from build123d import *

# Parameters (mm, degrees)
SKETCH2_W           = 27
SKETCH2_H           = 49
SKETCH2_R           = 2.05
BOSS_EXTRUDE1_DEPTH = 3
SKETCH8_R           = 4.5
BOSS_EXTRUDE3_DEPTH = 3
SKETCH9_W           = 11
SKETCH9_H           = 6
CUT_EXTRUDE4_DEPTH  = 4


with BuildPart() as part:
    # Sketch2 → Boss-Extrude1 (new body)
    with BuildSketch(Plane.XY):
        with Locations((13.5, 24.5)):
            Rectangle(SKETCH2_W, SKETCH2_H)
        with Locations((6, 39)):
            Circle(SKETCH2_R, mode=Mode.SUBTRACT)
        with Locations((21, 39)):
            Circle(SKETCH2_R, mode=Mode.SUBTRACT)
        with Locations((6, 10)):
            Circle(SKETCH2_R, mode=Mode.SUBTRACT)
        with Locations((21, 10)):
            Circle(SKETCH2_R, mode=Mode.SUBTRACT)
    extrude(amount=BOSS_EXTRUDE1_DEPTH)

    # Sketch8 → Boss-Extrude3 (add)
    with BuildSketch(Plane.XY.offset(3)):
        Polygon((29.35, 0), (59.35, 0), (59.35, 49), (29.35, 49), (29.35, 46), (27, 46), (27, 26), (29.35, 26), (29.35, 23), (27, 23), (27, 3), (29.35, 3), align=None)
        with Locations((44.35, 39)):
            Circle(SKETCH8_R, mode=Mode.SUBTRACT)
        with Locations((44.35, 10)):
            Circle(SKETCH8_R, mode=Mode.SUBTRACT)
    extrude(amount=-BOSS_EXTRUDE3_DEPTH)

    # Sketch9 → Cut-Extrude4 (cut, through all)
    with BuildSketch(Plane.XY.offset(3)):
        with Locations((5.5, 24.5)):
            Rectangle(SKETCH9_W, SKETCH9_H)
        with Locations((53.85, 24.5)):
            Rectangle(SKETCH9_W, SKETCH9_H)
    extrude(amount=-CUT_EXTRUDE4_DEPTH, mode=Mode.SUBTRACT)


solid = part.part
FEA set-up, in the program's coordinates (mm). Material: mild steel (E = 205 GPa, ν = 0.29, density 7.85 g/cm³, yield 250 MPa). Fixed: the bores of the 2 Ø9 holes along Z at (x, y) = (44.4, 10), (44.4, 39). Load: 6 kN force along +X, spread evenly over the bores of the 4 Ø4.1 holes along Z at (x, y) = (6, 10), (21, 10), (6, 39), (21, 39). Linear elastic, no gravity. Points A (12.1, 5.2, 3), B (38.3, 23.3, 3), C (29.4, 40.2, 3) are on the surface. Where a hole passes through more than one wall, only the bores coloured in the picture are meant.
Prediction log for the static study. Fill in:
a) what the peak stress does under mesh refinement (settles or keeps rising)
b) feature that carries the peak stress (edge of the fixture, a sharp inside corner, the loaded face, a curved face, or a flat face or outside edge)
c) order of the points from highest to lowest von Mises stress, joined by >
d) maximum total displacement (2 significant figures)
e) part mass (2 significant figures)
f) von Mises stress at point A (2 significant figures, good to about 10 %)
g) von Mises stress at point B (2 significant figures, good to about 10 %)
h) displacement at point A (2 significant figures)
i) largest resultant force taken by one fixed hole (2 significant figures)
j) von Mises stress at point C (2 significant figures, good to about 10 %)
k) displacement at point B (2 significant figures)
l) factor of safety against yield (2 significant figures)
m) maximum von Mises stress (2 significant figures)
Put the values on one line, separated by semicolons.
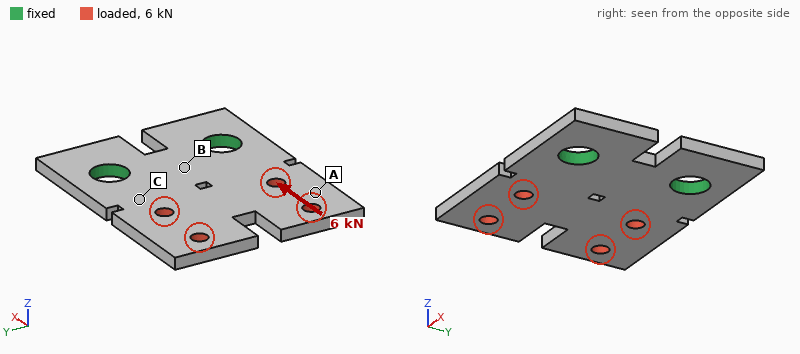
settles; the loaded face; C > A > B; 9.5 µm; 61 g; 33 MPa; 16 MPa; 7.6 µm; 3.0 kN; 52 MPa; 1.9 µm; 1.7; 150 MPa
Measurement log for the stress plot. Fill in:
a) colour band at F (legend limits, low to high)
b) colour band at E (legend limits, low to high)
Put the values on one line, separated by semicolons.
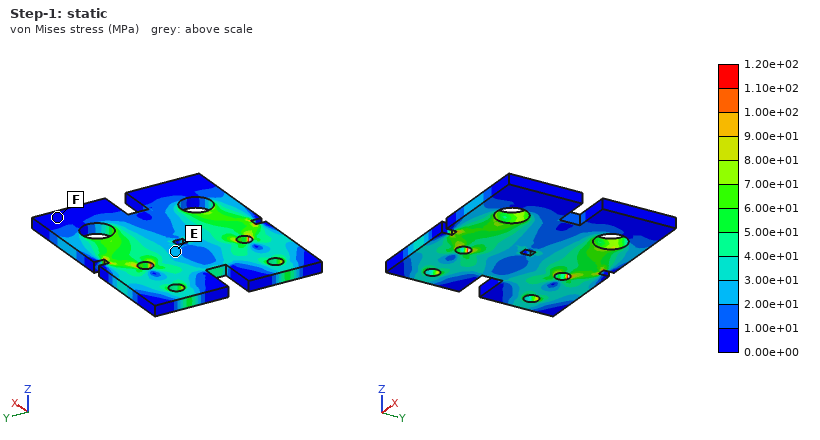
0.00e+00 to 1.00e+01 MPa; 2.00e+01 to 3.00e+01 MPa
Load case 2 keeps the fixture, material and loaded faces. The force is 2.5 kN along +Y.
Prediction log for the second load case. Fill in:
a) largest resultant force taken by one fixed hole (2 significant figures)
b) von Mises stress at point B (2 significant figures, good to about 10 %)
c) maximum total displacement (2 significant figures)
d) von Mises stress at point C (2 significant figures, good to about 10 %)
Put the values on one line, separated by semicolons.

2.4 kN; 30 MPa; 19 µm; 33 MPa
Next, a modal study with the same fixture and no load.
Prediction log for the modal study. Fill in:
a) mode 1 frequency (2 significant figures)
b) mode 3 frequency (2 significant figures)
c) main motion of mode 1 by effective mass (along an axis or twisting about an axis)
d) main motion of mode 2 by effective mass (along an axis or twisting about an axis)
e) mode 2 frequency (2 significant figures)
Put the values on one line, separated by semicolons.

1500 Hz; 7100 Hz; along Z; twisting about X; 2800 Hz
